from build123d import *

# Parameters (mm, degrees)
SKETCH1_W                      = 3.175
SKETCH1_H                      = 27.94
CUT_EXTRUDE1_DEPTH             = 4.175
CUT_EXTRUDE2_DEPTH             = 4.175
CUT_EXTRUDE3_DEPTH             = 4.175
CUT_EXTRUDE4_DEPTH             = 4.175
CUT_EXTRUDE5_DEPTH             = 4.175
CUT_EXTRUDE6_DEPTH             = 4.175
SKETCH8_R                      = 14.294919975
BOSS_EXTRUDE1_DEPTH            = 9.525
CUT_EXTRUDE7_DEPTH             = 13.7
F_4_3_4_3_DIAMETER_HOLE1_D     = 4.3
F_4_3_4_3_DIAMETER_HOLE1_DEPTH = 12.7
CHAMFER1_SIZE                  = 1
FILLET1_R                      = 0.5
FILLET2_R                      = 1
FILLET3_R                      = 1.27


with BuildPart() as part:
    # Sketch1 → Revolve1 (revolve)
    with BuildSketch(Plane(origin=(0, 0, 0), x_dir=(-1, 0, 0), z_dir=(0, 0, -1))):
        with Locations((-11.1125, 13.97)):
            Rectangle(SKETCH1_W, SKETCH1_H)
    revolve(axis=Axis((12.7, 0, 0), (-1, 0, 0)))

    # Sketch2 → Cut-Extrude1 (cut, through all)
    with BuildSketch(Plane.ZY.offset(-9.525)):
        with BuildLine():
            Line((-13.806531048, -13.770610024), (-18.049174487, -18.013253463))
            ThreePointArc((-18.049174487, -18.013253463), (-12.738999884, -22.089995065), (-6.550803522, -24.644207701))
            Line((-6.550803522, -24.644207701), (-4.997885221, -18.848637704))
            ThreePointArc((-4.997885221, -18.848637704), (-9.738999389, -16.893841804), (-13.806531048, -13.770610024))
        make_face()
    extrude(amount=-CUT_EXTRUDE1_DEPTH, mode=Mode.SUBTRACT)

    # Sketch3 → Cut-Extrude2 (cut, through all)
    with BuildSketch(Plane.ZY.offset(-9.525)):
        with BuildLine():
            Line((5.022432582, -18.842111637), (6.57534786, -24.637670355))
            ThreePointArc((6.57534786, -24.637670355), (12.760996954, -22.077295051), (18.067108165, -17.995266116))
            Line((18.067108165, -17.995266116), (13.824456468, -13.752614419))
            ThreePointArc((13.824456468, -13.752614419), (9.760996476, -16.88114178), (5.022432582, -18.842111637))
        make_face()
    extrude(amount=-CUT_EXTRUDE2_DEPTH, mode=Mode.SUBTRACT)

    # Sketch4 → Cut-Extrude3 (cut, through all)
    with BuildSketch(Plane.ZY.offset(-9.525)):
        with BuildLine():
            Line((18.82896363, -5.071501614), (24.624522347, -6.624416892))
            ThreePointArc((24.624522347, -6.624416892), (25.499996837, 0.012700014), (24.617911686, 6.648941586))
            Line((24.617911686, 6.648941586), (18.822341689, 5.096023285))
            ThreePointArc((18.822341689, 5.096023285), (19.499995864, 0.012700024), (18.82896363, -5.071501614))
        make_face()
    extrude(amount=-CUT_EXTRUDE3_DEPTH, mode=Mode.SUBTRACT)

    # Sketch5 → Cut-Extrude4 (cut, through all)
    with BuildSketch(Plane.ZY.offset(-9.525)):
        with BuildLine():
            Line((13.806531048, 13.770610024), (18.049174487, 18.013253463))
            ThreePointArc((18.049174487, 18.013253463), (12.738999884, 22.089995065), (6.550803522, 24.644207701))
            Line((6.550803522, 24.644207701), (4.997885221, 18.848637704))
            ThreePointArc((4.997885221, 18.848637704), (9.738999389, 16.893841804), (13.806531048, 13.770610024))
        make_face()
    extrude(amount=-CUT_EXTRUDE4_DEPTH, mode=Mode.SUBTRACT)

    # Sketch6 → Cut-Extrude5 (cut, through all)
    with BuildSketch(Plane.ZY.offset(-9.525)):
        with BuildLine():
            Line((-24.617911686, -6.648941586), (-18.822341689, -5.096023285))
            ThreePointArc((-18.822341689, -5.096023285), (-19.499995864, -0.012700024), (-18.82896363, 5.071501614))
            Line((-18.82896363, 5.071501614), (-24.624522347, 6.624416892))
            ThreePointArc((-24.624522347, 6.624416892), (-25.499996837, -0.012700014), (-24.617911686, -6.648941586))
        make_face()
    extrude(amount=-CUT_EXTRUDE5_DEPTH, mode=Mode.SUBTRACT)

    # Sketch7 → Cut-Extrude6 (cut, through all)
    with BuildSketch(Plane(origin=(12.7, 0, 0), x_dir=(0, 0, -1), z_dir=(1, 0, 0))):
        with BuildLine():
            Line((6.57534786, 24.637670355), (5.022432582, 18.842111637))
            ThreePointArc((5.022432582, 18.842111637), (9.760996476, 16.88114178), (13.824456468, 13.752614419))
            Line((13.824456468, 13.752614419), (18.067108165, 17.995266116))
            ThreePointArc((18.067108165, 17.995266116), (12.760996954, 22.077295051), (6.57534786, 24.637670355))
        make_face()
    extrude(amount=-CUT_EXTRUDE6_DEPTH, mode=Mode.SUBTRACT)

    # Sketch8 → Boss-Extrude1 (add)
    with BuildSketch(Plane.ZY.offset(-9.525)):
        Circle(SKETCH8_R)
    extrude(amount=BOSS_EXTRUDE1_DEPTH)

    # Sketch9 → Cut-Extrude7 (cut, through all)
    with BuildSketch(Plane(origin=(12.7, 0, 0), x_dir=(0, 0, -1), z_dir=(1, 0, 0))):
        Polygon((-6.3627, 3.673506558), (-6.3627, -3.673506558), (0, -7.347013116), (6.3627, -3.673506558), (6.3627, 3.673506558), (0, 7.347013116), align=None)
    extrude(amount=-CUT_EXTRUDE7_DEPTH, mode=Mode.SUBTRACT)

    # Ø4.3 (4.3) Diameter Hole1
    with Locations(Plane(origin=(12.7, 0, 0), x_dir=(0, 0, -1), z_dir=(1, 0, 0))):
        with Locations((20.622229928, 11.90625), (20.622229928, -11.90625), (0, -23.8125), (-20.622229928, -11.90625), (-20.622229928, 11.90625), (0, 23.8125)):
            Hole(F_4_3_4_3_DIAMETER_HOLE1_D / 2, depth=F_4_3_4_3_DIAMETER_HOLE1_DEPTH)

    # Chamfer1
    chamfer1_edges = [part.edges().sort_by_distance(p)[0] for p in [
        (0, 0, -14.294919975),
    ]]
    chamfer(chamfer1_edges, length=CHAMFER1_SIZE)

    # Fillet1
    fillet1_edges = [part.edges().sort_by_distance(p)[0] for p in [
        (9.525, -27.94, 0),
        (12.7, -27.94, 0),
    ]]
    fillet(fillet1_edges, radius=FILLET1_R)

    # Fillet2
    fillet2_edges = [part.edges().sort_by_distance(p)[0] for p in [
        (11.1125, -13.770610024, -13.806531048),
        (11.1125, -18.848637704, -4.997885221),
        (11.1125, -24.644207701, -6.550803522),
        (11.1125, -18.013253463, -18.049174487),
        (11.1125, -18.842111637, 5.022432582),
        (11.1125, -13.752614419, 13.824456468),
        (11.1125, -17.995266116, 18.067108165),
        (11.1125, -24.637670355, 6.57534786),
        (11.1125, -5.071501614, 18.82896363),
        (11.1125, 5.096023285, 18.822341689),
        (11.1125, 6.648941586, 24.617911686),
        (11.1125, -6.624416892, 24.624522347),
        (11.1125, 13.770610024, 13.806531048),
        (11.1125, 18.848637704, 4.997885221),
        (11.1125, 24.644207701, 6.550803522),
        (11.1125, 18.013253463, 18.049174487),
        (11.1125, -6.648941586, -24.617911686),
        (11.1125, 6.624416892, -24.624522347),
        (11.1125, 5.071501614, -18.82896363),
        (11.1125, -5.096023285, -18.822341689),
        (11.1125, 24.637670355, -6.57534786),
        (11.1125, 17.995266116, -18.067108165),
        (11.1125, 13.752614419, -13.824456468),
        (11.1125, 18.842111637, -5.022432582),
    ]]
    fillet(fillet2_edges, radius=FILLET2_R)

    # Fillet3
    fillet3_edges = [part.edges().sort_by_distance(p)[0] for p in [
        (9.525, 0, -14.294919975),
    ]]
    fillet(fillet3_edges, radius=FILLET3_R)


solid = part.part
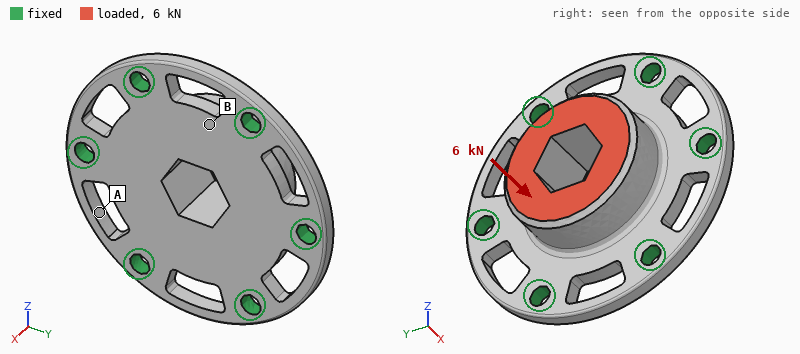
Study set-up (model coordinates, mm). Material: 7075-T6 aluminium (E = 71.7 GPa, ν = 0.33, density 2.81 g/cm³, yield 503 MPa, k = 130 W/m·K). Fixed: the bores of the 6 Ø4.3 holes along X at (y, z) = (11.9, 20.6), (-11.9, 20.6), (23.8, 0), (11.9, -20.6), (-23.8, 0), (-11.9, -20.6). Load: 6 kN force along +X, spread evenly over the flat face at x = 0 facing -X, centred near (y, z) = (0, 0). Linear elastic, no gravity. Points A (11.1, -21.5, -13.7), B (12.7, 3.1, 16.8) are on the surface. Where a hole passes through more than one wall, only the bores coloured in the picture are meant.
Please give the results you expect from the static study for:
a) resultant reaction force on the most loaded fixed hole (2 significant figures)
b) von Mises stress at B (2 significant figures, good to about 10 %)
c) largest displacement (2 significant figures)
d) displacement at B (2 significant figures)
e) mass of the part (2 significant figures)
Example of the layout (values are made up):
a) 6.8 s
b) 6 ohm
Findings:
a) 1.2 kN
b) 63 MPa
c) 46 µm
d) 31 µm
e) 29 g
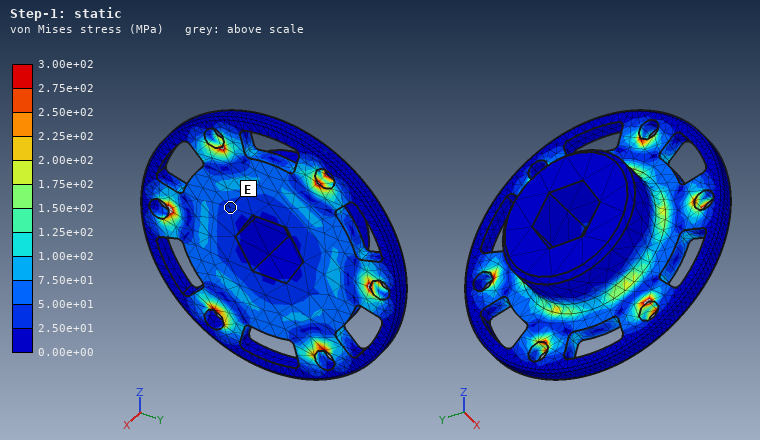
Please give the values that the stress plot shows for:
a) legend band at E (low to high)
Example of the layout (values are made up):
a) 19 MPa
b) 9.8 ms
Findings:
a) 2.50e+01 to 5.00e+01 MPa
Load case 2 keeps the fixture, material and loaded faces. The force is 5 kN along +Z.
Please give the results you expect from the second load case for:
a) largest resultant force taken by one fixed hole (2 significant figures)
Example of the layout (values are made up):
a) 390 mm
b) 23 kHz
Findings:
a) 1.4 kN
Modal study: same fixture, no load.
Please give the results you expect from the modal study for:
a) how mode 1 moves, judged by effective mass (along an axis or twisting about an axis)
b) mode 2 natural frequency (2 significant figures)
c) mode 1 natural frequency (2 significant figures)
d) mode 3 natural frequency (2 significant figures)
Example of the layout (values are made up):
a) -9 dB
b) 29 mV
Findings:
a) along X
b) 18 kHz
c) 13 kHz
d) 18 kHz
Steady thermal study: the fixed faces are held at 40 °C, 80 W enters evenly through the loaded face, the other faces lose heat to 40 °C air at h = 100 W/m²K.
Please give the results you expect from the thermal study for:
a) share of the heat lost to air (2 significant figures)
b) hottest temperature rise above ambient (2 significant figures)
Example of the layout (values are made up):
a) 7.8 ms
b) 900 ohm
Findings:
a) 10 %
b) 38 K
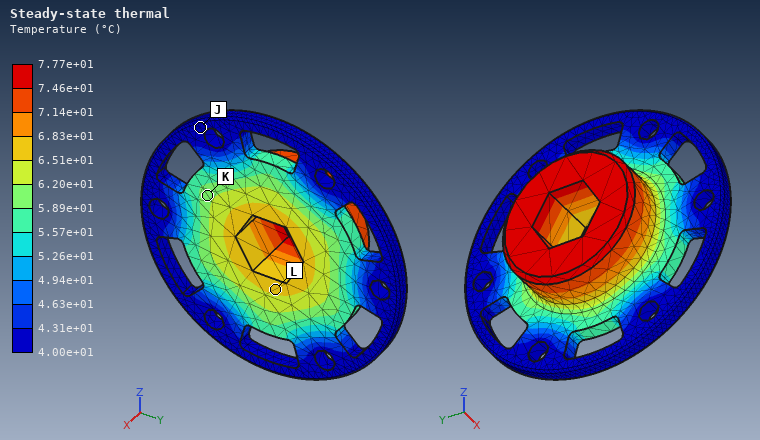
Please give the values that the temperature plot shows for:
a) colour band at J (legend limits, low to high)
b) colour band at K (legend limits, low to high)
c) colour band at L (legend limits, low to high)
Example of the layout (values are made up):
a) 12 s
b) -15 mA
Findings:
a) 4.00e+01 to 4.31e+01 °C
b) 5.89e+01 to 6.20e+01 °C
c) 6.51e+01 to 6.83e+01 °C
